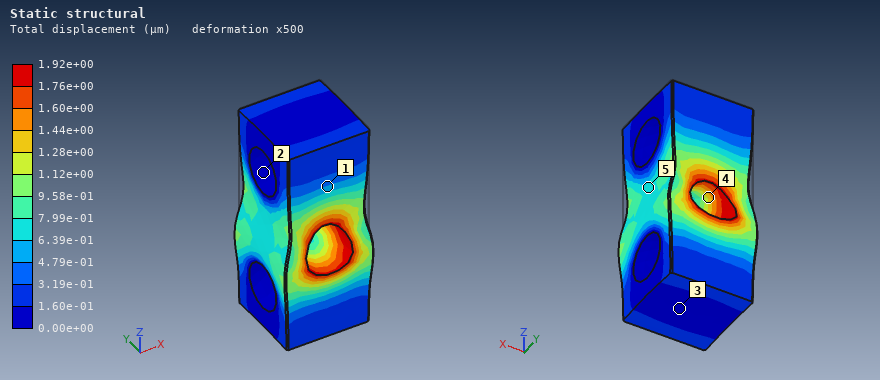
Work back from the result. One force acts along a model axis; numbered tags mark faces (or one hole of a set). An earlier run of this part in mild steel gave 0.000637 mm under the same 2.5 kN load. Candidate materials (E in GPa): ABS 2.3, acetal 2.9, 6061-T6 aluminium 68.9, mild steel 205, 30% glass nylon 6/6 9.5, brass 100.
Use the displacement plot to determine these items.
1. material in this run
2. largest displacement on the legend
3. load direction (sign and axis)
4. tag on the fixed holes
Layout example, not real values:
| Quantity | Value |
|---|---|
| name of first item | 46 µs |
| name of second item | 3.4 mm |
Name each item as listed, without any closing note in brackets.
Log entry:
| Quantity | Value |
|---|---|
| material in this run | 6061-T6 aluminium |
| largest displacement on the legend | 1.92e+00 µm |
| load direction | -Z |
| tag on the fixed holes | 2 |
